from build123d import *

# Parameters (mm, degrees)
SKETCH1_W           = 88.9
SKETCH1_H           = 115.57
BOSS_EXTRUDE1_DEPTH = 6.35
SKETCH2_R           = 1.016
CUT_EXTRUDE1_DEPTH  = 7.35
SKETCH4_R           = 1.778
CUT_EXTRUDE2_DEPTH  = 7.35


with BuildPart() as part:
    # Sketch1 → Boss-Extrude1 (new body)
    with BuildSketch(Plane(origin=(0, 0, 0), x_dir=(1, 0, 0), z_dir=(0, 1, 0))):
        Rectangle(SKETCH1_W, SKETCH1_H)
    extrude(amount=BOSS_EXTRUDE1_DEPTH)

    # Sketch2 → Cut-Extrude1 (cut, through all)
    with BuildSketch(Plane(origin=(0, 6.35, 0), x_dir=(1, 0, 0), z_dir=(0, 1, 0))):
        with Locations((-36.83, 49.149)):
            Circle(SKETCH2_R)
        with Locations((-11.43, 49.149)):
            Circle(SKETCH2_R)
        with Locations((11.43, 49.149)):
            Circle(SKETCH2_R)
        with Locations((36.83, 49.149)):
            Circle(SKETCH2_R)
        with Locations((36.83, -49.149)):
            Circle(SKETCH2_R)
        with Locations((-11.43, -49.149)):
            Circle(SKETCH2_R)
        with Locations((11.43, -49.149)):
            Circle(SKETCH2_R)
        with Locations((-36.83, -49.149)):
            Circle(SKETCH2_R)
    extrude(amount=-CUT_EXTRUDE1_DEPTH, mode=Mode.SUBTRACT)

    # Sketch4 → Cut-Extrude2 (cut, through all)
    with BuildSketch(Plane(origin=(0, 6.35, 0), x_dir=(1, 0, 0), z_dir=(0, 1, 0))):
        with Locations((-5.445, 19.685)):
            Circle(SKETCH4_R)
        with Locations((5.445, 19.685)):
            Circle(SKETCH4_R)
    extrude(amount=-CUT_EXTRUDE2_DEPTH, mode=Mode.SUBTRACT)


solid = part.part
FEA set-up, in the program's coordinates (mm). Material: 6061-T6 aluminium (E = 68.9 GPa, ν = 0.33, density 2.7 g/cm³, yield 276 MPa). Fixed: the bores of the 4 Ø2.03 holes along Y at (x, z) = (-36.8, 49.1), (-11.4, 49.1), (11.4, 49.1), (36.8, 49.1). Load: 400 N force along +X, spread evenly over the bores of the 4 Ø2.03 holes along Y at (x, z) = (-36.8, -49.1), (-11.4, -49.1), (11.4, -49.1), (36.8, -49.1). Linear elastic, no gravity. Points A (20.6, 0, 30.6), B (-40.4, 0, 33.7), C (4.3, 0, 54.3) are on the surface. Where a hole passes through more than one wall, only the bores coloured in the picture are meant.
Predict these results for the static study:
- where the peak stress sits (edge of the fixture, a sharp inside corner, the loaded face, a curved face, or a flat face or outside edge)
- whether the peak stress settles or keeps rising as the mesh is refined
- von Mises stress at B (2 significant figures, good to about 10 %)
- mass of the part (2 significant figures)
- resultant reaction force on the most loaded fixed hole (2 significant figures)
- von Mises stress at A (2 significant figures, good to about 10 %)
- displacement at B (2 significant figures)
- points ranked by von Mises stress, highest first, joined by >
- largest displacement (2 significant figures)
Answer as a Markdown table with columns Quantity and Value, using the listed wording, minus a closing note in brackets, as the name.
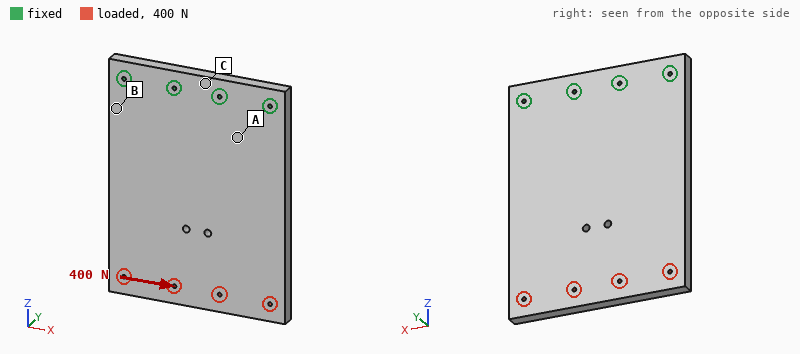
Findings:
| Quantity | Value |
|---|---|
| where the peak stress sits | edge of the fixture |
| whether the peak stress settles or keeps rising as the mesh is refined | keeps rising |
| von Mises stress at B | 3.8 MPa |
| mass of the part | 180 g |
| resultant reaction force on the most loaded fixed hole | 500 N |
| von Mises stress at A | 2.0 MPa |
| displacement at B | 1.8 µm |
| points ranked by von Mises stress, highest first, joined by > | B > A > C |
| largest displacement | 11 µm |
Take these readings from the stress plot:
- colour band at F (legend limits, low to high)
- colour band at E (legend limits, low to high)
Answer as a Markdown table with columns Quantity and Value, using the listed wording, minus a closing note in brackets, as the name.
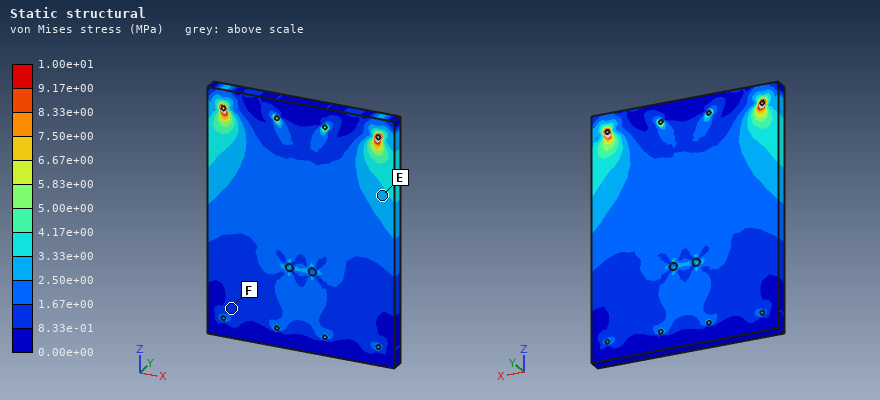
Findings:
| Quantity | Value |
|---|---|
| colour band at F | 8.33e-01 to 1.67e+00 MPa |
| colour band at E | 2.50e+00 to 3.33e+00 MPa |
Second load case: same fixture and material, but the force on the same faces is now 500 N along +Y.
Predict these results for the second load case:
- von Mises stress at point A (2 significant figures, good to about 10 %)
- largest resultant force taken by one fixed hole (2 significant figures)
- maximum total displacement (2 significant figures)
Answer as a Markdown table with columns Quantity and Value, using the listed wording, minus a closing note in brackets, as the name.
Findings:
| Quantity | Value |
|---|---|
| von Mises stress at point A | 61 MPa |
| largest resultant force taken by one fixed hole | 290 N |
| maximum total displacement | 1.5 mm |
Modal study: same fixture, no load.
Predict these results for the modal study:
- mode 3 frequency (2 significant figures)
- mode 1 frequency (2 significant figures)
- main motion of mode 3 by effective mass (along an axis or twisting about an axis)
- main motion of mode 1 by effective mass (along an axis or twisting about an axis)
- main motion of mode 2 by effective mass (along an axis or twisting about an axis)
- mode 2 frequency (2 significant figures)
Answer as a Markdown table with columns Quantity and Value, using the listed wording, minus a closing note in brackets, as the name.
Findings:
| Quantity | Value |
|---|---|
| mode 3 frequency | 2600 Hz |
| mode 1 frequency | 430 Hz |
| main motion of mode 3 by effective mass | along Y |
| main motion of mode 1 by effective mass | along Y |
| main motion of mode 2 by effective mass | twisting about Z |
| mode 2 frequency | 1200 Hz |
